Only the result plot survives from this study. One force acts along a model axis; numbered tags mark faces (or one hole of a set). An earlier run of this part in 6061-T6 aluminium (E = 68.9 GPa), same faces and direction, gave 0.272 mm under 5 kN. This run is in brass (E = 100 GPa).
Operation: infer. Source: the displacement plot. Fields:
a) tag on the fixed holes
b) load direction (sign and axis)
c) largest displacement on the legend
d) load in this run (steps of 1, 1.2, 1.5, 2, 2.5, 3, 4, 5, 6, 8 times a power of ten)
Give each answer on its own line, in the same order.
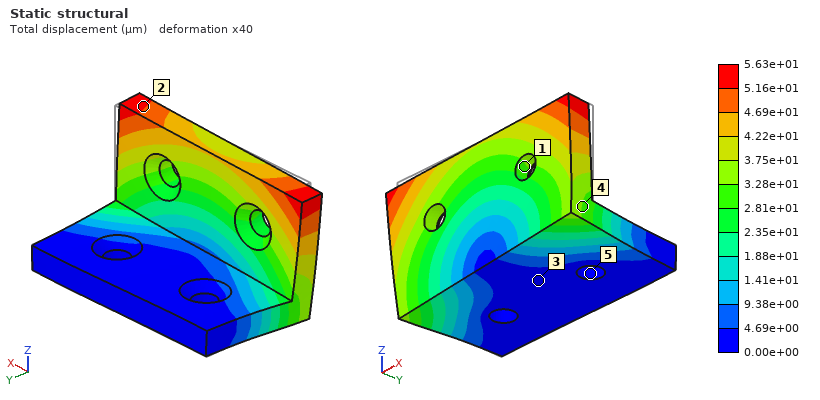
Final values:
5
-X
5.63e+01 µm
1.5 kN
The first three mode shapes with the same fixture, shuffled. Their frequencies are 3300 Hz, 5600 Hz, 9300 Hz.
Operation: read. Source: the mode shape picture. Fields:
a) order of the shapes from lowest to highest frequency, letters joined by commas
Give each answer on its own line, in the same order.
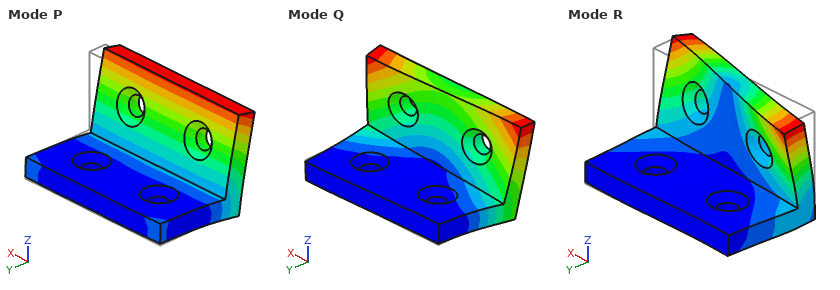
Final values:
P, Q, R
